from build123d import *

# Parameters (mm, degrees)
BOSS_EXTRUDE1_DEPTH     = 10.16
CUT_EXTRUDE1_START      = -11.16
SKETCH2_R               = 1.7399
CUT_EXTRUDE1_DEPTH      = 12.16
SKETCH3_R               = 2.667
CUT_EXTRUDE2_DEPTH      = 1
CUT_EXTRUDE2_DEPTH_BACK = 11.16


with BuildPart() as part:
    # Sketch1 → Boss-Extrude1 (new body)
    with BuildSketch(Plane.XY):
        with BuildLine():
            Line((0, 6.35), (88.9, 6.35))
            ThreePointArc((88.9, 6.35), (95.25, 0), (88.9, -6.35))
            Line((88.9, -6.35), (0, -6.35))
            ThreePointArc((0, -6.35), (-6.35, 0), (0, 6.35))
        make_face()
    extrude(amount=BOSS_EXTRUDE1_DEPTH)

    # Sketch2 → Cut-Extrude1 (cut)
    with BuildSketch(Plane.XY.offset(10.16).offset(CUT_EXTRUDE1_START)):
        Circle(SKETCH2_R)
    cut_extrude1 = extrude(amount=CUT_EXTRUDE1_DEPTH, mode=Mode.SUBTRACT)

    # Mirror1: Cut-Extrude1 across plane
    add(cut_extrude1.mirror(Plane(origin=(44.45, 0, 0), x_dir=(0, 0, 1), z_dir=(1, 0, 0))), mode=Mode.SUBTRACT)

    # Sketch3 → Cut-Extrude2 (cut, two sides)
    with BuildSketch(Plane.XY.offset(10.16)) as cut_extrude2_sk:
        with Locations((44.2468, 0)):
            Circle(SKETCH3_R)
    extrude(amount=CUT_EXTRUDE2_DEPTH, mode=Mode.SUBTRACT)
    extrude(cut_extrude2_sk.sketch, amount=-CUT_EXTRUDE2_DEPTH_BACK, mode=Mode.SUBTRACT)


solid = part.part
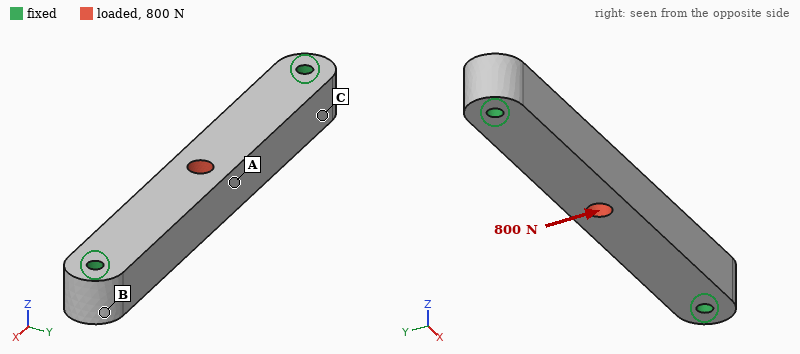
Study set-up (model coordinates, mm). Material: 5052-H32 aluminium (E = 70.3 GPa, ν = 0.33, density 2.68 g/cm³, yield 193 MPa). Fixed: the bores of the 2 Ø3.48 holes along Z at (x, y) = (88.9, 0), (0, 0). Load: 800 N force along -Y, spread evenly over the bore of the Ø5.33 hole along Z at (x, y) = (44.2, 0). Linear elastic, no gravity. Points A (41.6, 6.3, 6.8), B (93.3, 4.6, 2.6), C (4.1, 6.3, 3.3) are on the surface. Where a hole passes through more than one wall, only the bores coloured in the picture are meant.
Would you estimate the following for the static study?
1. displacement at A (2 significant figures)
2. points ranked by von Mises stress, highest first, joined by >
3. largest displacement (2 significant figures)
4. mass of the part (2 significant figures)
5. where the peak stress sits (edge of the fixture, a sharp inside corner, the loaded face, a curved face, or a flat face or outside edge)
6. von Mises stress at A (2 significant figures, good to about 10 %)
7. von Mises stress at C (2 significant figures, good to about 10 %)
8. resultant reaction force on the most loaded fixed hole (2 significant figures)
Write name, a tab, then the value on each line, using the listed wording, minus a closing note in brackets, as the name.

displacement at A	42 µm
points ranked by von Mises stress, highest first, joined by >	A > C > B
largest displacement	43 µm
mass of the part	33 g
where the peak stress sits	edge of the fixture
von Mises stress at A	37 MPa
von Mises stress at C	20 MPa
resultant reaction force on the most loaded fixed hole	400 N
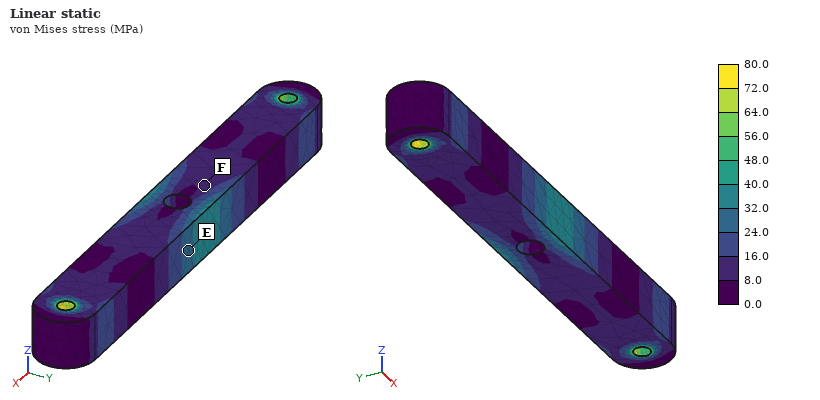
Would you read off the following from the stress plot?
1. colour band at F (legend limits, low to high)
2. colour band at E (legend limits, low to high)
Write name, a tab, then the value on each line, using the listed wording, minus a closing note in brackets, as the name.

colour band at F	8.0 to 16.0 MPa
colour band at E	24.0 to 32.0 MPa
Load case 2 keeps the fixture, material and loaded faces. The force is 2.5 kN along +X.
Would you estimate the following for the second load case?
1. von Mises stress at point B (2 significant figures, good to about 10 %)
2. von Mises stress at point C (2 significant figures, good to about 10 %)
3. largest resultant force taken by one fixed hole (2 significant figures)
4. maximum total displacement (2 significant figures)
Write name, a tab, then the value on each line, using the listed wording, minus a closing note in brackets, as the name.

von Mises stress at point B	3.1 MPa
von Mises stress at point C	5.6 MPa
largest resultant force taken by one fixed hole	1.3 kN
maximum total displacement	6.6 µm
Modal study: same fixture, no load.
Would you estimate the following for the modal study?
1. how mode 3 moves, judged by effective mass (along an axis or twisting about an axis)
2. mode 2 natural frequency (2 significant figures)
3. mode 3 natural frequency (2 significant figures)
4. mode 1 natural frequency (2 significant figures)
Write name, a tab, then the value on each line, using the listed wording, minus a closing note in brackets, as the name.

how mode 3 moves, judged by effective mass	twisting about Y
mode 2 natural frequency	6100 Hz
mode 3 natural frequency	15 kHz
mode 1 natural frequency	6100 Hz
